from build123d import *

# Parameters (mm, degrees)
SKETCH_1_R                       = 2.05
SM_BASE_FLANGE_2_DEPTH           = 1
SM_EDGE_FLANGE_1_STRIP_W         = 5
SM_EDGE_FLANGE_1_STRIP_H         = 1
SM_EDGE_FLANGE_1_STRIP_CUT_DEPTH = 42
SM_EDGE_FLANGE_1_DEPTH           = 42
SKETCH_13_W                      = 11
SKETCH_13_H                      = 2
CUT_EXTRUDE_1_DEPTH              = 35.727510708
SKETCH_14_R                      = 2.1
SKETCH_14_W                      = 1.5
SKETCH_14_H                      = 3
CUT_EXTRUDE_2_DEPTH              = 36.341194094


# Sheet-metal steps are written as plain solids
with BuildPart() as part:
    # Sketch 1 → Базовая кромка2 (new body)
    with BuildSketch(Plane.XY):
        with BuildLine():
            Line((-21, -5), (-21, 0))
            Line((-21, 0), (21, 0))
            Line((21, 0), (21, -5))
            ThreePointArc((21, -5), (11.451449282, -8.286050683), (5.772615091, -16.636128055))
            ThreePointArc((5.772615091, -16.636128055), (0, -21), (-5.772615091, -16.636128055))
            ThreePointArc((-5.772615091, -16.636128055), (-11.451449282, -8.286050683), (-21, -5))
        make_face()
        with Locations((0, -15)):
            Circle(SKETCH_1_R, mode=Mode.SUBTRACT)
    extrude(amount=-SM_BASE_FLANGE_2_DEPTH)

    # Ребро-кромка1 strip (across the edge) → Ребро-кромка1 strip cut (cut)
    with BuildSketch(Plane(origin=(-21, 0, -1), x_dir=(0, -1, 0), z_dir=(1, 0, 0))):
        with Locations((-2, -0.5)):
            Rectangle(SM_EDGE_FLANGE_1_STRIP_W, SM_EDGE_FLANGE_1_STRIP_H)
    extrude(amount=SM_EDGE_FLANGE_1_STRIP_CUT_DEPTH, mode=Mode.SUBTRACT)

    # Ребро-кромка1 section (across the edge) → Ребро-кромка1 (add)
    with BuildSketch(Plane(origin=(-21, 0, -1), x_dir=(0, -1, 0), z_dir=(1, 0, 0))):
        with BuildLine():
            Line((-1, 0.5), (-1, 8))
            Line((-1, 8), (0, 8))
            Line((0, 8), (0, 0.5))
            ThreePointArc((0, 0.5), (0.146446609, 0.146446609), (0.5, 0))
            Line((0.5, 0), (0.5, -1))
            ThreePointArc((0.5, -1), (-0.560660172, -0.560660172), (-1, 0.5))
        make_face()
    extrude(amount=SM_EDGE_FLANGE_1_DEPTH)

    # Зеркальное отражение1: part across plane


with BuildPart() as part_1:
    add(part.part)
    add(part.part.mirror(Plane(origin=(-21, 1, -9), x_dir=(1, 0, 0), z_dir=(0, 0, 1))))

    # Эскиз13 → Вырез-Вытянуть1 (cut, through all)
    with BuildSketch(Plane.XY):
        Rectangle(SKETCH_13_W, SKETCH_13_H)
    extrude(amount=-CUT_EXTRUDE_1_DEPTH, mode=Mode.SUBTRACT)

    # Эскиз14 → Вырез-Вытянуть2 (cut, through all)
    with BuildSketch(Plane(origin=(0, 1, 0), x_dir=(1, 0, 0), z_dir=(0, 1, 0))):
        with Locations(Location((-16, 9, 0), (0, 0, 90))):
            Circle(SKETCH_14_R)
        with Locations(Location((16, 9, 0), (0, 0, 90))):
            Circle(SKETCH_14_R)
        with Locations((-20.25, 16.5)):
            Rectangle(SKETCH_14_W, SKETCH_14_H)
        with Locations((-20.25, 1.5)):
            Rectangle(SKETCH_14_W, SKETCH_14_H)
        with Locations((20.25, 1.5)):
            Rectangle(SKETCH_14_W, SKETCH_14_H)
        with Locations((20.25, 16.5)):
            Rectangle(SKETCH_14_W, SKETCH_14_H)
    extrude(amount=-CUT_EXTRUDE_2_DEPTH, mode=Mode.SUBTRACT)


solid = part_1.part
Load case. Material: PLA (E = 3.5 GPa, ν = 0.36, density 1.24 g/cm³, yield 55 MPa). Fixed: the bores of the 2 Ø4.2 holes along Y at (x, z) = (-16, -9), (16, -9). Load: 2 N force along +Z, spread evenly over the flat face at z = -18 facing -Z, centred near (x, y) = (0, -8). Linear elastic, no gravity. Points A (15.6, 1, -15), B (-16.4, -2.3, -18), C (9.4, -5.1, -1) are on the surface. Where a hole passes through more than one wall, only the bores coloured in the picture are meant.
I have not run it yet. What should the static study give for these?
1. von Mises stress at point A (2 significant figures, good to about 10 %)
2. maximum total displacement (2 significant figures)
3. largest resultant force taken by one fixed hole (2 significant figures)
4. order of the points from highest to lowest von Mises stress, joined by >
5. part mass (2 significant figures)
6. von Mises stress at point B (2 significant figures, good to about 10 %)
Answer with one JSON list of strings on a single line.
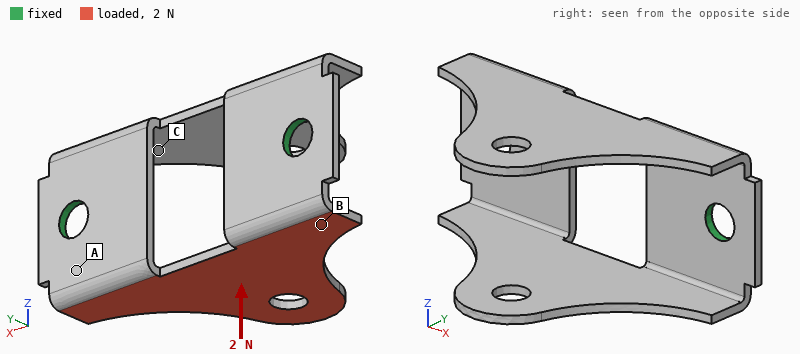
["2.7 MPa", "0.53 mm", "1.0 N", "A > B > C", "1.7 g", "1.7 MPa"]
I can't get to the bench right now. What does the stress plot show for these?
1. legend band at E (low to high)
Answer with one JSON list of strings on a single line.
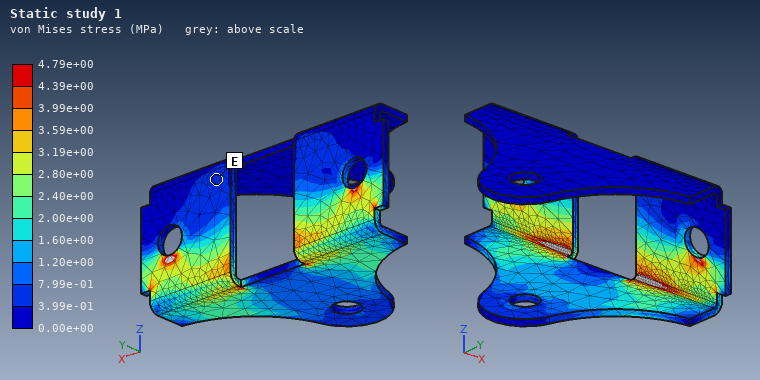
["3.99e-01 to 7.99e-01 MPa"]
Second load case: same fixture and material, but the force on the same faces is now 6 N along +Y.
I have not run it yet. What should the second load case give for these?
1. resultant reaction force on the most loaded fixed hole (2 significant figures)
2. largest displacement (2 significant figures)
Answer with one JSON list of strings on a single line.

["3.5 N", "0.48 mm"]
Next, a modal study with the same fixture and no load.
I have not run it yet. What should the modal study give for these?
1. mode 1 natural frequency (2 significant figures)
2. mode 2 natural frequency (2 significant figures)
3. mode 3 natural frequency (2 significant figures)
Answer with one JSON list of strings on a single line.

["580 Hz", "580 Hz", "1800 Hz"]
